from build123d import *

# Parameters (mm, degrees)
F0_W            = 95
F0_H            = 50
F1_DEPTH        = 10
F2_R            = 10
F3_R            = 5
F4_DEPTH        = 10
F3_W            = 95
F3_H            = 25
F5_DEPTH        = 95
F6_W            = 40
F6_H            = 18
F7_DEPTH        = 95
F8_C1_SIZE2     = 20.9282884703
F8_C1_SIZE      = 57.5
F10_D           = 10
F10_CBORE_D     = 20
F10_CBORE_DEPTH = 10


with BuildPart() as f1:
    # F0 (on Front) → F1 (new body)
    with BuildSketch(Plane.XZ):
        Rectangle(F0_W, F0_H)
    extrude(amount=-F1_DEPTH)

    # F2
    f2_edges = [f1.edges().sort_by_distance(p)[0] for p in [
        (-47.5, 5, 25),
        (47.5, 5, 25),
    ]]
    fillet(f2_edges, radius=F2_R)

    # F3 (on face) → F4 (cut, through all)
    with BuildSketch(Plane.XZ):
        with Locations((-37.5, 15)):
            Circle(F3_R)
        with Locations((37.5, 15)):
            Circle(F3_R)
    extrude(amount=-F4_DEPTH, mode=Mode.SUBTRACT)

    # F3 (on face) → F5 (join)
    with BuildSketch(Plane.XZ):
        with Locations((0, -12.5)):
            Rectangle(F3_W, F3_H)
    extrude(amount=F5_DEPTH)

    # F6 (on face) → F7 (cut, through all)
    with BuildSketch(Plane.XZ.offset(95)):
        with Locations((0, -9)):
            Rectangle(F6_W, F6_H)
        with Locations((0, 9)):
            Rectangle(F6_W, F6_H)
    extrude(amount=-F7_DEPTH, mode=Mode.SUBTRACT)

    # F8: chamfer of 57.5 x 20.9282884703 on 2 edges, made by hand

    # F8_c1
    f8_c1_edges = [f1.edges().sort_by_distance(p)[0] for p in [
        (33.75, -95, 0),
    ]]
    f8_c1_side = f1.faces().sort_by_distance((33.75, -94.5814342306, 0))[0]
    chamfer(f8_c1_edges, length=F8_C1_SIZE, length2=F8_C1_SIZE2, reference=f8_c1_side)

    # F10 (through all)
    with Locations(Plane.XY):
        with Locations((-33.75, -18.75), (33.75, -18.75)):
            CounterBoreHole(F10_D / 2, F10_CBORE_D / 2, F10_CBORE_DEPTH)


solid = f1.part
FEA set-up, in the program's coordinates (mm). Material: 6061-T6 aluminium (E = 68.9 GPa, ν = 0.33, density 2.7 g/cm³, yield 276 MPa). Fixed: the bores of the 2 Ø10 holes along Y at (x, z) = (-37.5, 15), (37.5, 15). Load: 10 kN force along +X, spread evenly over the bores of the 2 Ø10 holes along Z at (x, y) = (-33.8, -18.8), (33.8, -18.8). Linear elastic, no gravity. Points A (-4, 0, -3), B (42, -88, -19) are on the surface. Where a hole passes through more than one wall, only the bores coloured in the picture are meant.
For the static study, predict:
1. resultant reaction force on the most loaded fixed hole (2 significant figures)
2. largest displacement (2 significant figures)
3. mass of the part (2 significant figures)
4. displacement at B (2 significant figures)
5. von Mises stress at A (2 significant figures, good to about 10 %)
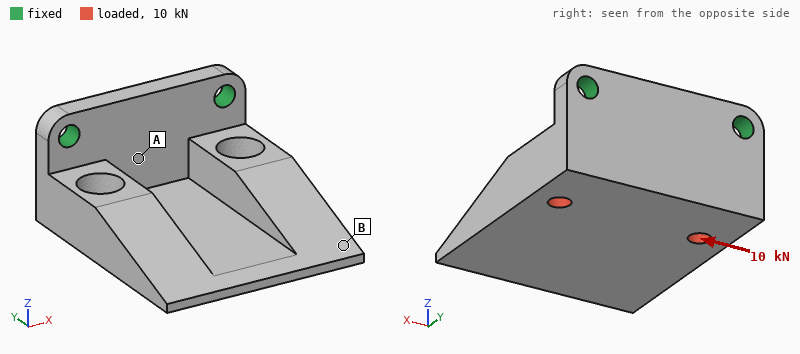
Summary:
6.9 kN
0.17 mm
430 g
0.16 mm
31 MPa
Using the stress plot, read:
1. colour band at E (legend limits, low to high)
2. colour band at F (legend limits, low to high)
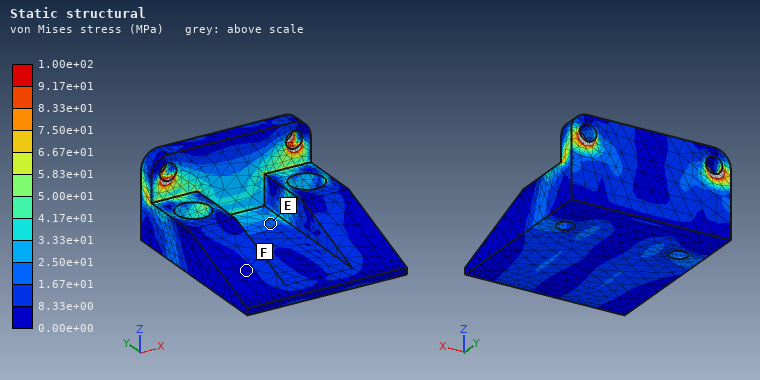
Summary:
1.67e+01 to 2.50e+01 MPa
0.00e+00 to 8.33e+00 MPa
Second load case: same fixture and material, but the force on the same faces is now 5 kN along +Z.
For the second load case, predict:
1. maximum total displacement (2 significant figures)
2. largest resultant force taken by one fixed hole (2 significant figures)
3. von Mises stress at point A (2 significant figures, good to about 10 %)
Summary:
0.58 mm
2.5 kN
29 MPa
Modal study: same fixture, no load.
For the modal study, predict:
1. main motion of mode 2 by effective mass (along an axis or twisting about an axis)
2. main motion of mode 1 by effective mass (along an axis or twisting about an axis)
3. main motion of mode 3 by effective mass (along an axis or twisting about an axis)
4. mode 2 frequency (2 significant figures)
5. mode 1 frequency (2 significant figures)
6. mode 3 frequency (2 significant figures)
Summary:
along X
along Z
along X
1700 Hz
700 Hz
3200 Hz
